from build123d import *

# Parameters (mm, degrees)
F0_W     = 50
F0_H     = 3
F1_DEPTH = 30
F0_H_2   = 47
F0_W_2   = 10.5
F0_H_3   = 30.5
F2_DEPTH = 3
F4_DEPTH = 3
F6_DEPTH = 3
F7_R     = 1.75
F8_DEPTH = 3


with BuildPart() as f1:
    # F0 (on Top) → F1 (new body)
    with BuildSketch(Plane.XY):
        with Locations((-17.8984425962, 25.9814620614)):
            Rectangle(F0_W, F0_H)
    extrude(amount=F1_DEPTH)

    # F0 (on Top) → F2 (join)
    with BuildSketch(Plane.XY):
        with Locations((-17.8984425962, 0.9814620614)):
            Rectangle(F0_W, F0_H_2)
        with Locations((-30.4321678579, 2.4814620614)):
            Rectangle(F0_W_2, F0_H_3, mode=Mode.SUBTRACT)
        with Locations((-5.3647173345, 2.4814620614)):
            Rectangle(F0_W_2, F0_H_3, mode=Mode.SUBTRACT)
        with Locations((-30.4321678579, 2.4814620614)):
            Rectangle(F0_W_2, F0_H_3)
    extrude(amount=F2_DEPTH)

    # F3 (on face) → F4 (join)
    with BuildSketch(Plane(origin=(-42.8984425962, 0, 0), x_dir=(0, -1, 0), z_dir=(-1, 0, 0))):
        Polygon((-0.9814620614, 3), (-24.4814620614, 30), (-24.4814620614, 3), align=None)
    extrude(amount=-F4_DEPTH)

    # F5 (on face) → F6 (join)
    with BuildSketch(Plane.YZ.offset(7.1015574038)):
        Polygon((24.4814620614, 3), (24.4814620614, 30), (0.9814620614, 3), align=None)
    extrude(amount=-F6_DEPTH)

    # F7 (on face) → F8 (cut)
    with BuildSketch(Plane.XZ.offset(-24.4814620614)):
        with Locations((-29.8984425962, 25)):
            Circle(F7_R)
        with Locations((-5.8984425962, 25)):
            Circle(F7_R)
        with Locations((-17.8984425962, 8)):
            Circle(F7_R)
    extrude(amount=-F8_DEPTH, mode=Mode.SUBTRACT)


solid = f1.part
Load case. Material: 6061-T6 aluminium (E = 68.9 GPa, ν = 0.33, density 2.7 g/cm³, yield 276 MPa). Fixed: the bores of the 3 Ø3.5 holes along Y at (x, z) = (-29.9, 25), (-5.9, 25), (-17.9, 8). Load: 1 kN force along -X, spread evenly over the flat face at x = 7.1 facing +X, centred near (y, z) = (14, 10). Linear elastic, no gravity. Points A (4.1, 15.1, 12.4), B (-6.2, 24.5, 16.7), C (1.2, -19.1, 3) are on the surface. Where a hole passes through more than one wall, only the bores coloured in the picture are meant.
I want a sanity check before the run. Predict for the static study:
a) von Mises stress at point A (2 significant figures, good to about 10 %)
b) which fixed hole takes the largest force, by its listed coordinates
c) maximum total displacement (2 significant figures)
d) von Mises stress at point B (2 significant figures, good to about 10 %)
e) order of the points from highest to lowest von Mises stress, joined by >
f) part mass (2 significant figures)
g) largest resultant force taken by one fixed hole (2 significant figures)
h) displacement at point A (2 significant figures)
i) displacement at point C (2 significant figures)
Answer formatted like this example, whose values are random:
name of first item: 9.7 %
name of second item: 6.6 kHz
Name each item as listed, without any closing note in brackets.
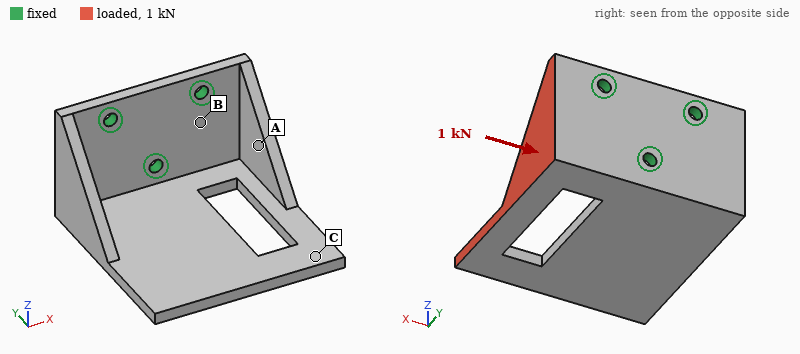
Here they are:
von Mises stress at point A: 34 MPa
which fixed hole takes the largest force, by its listed coordinates: (-17.9, 8)
maximum total displacement: 0.36 mm
von Mises stress at point B: 60 MPa
order of the points from highest to lowest von Mises stress, joined by >: B > A > C
part mass: 33 g
largest resultant force taken by one fixed hole: 680 N
displacement at point A: 0.13 mm
displacement at point C: 0.29 mm
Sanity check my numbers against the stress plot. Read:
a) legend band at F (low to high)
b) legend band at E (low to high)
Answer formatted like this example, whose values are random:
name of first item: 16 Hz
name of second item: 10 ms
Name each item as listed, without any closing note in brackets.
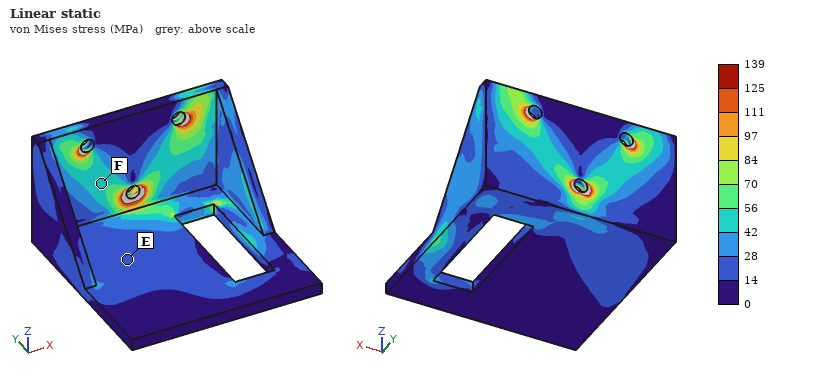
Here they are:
legend band at F: 42 to 56 MPa
legend band at E: 14 to 28 MPa
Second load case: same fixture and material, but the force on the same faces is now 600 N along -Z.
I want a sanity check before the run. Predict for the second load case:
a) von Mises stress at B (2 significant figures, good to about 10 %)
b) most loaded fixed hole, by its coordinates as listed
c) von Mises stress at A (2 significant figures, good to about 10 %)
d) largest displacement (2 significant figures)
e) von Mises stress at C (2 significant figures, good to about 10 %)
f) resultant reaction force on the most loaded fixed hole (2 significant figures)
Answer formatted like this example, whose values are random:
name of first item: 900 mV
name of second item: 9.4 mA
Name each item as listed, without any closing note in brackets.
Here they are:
von Mises stress at B: 37 MPa
most loaded fixed hole, by its coordinates as listed: (-5.9, 25)
von Mises stress at A: 17 MPa
largest displacement: 0.30 mm
von Mises stress at C: 14 MPa
resultant reaction force on the most loaded fixed hole: 710 N
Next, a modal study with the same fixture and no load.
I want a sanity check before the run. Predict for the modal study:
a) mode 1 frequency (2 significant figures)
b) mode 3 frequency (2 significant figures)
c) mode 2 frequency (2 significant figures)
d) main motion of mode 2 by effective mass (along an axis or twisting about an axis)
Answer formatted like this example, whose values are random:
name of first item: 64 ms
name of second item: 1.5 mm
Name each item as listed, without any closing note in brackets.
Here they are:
mode 1 frequency: 1500 Hz
mode 3 frequency: 4100 Hz
mode 2 frequency: 1700 Hz
main motion of mode 2 by effective mass: along Z
